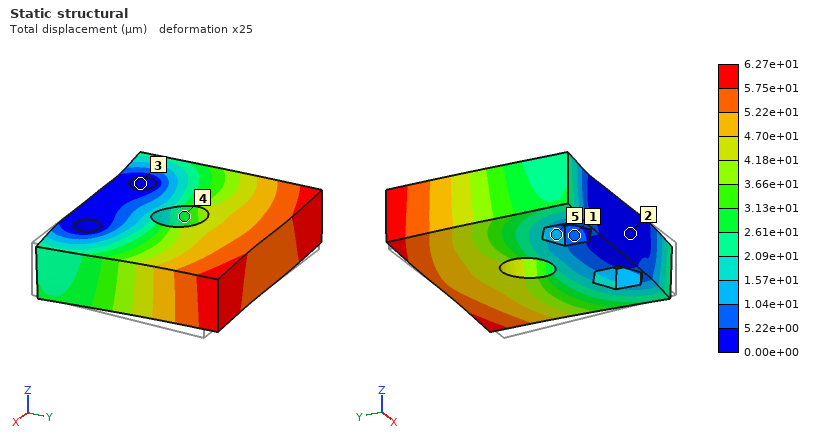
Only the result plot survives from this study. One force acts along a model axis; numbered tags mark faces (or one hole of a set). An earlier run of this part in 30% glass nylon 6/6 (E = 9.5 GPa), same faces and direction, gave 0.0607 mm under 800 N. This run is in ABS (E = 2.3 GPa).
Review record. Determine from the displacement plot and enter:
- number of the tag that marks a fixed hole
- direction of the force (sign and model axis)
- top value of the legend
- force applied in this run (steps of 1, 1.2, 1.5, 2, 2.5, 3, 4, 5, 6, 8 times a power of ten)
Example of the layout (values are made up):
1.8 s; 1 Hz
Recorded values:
3; -X; 6.27e+01 µm; 200 N
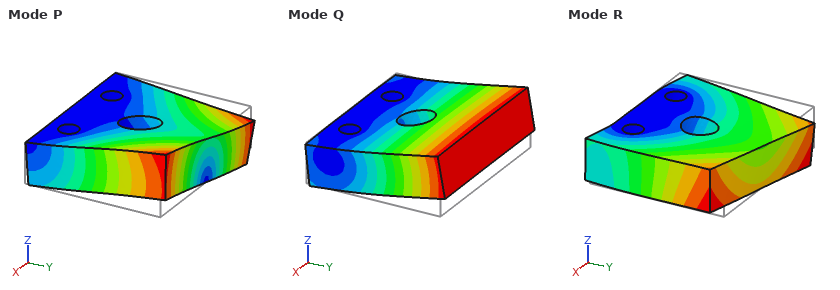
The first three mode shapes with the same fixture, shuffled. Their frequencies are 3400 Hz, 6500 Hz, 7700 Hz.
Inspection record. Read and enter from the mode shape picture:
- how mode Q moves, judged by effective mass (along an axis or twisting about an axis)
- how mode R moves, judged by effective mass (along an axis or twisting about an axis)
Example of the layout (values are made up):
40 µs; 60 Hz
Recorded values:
along Z; along X
